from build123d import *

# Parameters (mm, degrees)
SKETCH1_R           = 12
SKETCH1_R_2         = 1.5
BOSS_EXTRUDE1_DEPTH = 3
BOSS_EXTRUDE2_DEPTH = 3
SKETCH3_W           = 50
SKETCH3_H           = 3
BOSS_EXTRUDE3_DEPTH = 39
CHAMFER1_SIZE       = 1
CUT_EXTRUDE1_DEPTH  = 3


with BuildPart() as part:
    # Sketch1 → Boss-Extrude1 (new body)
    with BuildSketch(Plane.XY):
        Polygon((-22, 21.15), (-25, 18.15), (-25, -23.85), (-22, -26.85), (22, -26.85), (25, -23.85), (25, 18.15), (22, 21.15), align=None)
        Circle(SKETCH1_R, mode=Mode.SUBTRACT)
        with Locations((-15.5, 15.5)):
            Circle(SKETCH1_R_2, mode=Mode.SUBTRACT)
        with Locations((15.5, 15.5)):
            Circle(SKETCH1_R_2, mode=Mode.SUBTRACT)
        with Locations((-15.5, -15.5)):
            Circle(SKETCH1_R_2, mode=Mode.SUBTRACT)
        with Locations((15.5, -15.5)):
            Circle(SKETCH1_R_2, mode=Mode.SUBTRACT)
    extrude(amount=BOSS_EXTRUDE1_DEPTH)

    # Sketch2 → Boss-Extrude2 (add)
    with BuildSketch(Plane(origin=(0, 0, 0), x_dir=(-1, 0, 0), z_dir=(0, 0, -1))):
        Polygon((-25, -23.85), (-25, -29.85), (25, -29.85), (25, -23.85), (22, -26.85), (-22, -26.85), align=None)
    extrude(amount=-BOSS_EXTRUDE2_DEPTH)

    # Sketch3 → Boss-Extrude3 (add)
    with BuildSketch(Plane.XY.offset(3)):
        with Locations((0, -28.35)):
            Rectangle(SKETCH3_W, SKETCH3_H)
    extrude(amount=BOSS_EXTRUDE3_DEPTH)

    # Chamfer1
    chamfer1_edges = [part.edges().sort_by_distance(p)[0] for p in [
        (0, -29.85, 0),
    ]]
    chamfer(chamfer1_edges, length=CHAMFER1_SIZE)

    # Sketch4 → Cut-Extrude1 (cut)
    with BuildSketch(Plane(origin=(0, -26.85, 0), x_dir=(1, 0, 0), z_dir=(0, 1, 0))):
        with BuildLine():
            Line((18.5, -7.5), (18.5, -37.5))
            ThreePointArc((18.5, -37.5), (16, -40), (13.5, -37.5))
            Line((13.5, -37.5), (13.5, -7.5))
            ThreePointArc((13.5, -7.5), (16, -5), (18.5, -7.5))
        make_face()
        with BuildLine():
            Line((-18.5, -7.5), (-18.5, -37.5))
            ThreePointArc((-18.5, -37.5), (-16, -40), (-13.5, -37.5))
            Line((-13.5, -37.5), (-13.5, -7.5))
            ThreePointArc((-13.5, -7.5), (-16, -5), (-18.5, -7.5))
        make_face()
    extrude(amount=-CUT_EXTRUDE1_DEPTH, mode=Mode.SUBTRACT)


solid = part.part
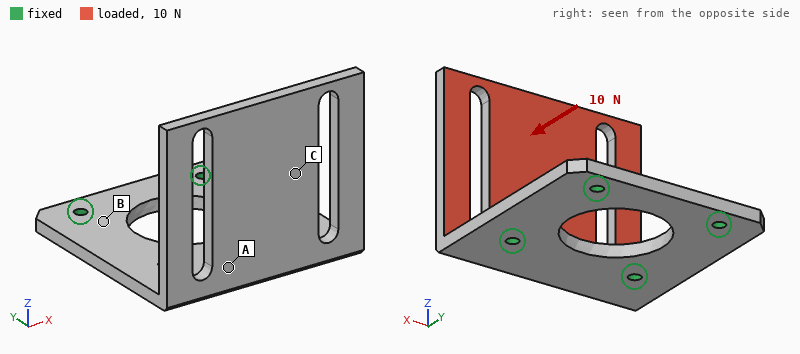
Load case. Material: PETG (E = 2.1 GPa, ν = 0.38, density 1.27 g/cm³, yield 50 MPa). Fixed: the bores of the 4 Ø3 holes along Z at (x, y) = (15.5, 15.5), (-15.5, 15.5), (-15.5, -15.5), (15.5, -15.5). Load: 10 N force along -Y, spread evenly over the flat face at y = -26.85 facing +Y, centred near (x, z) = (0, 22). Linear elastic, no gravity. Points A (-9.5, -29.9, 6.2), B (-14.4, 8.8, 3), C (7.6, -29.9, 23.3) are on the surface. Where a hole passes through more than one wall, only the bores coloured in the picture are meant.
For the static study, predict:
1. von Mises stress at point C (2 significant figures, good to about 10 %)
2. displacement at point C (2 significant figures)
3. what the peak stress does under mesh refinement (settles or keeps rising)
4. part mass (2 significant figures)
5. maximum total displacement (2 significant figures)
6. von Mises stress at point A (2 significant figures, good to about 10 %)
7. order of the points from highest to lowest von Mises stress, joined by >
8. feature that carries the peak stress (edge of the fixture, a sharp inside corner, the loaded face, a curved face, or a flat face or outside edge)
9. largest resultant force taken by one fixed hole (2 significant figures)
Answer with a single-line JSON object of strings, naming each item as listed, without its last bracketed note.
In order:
{"von Mises stress at point C": "0.76 MPa", "displacement at point C": "0.42 mm", "what the peak stress does under mesh refinement": "keeps rising", "part mass": "14 g", "maximum total displacement": "0.86 mm", "von Mises stress at point A": "2.4 MPa", "order of the points from highest to lowest von Mises stress, joined by >": "A > C > B", "feature that carries the peak stress": "edge of the fixture", "largest resultant force taken by one fixed hole": "5.1 N"}
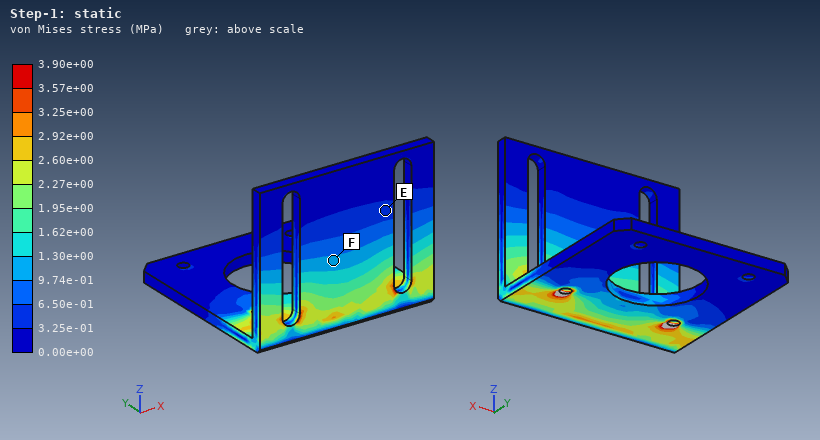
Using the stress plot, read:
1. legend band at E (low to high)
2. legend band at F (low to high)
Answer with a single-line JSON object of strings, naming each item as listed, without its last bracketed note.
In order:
{"legend band at E": "3.25e-01 to 6.50e-01 MPa", "legend band at F": "9.74e-01 to 1.30e+00 MPa"}
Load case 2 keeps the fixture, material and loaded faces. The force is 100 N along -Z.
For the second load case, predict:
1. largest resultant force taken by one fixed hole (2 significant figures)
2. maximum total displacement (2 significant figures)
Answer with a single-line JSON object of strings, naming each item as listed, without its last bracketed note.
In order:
{"largest resultant force taken by one fixed hole": "53 N", "maximum total displacement": "0.97 mm"}
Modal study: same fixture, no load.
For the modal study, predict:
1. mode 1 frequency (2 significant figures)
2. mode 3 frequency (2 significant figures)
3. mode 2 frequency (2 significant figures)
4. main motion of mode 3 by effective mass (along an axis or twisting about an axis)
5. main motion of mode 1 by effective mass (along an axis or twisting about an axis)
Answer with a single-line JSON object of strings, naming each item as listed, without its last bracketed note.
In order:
{"mode 1 frequency": "270 Hz", "mode 3 frequency": "880 Hz", "mode 2 frequency": "610 Hz", "main motion of mode 3 by effective mass": "along X", "main motion of mode 1 by effective mass": "along Y"}
